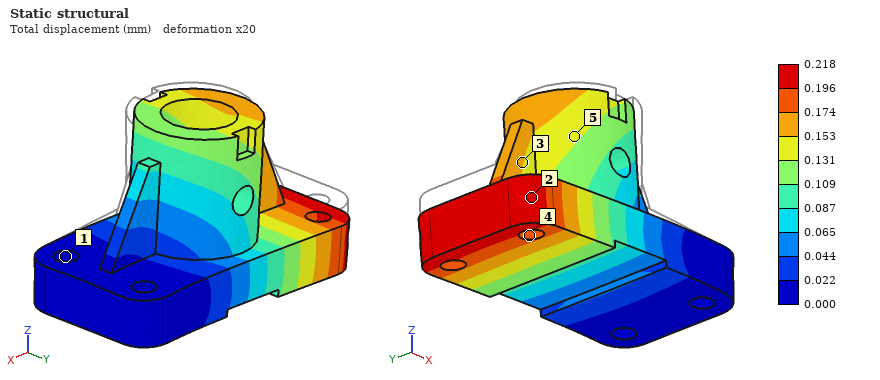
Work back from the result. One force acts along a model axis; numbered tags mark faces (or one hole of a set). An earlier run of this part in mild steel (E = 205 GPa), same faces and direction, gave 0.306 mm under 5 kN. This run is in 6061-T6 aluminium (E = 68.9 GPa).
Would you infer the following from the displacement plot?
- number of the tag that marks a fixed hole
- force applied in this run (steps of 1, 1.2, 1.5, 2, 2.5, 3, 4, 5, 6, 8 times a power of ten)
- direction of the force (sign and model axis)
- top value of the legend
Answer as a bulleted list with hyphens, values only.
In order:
- 1
- 1.2 kN
- -Z
- 0.218 mm
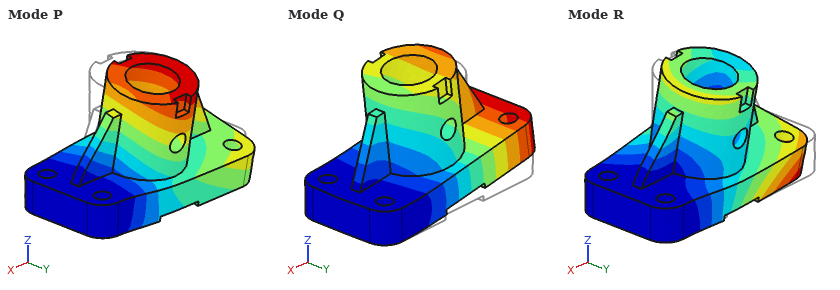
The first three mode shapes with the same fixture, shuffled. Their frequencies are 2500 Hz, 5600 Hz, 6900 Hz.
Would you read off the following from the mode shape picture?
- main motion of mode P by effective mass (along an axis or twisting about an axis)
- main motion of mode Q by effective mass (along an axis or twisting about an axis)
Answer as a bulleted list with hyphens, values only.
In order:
- along Y
- along Z
